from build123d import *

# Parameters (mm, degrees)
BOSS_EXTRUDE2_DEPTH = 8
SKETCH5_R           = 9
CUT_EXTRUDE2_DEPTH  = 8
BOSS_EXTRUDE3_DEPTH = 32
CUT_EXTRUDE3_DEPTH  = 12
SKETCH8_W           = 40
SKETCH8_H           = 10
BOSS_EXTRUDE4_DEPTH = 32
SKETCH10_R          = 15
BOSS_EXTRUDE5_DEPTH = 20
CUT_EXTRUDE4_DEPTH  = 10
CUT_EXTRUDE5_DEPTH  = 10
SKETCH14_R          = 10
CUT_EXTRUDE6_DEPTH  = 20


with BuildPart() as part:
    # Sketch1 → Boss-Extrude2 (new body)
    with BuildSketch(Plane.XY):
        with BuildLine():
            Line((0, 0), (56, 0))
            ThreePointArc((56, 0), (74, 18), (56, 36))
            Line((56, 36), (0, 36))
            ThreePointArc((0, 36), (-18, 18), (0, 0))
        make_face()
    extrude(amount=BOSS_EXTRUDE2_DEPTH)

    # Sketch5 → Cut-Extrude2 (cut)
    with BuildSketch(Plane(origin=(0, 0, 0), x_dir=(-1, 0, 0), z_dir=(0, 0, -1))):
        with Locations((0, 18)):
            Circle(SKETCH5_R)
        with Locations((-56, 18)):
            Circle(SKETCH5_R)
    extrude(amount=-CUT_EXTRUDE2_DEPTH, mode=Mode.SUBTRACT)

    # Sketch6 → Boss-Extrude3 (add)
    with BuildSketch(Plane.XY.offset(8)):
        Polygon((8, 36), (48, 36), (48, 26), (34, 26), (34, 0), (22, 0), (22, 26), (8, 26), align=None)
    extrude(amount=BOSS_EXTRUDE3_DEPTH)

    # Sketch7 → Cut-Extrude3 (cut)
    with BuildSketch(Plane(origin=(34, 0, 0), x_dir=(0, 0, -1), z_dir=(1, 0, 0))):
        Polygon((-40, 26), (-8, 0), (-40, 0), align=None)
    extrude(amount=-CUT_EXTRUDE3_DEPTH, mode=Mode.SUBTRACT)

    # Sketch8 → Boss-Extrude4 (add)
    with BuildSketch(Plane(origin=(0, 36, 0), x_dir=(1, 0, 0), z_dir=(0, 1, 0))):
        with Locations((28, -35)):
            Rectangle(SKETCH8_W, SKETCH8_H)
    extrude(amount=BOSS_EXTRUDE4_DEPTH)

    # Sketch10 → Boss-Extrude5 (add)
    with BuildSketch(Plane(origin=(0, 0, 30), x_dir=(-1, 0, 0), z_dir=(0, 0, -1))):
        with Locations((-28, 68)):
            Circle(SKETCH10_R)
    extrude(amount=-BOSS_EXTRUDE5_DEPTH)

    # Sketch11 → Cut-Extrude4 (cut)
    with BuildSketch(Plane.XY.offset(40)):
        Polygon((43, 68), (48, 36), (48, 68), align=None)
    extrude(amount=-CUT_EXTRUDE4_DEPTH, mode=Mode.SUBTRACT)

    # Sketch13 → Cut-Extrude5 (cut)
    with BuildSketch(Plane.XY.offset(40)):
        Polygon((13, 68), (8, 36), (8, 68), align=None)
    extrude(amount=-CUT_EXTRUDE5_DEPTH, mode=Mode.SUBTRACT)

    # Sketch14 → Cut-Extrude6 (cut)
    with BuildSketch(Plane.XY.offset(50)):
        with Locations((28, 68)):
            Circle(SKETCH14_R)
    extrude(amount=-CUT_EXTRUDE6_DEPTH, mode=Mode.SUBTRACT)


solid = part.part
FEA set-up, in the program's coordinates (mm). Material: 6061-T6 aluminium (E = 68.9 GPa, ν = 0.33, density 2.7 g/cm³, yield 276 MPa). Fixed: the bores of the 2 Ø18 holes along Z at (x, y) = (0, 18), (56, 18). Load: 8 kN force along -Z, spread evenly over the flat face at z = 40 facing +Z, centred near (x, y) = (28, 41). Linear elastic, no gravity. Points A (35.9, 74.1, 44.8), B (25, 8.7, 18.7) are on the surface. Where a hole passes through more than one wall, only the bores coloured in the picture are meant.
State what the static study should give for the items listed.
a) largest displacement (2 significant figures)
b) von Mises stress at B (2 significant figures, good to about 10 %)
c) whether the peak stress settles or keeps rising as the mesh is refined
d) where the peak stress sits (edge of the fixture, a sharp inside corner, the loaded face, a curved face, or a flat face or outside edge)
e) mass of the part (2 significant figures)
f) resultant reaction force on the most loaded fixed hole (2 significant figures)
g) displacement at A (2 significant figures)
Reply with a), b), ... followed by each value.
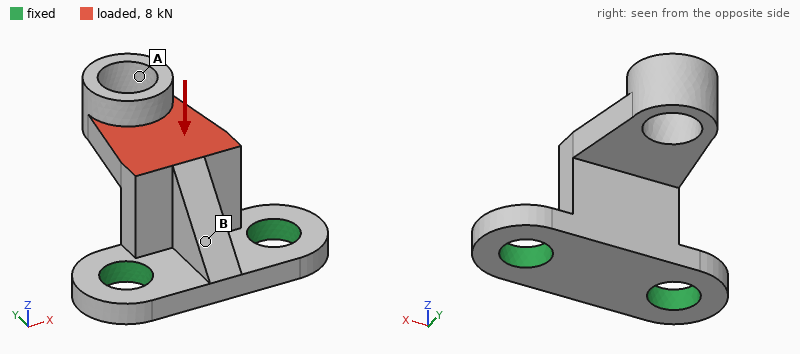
a) 0.55 mm
b) 43 MPa
c) keeps rising
d) edge of the fixture
e) 140 g
f) 4.4 kN
g) 0.46 mm
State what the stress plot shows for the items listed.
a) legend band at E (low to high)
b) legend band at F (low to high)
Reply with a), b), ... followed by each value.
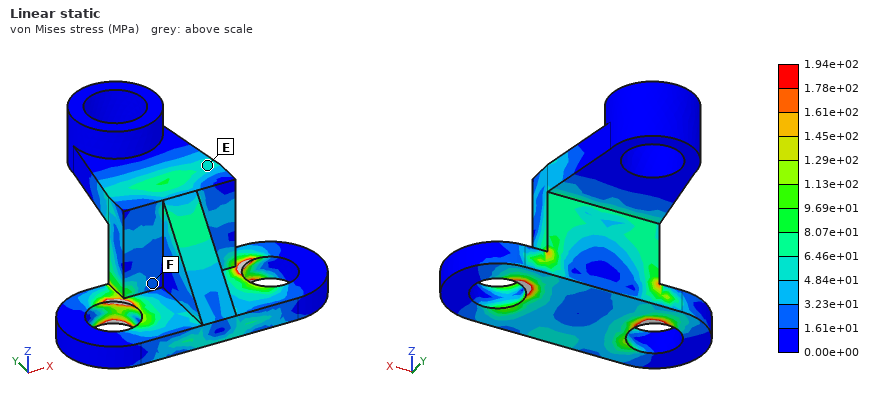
a) 4.84e+01 to 6.46e+01 MPa
b) 1.61e+01 to 3.23e+01 MPa
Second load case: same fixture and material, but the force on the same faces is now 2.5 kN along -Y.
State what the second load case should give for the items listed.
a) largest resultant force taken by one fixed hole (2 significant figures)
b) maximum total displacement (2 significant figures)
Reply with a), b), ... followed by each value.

a) 1.3 kN
b) 0.25 mm
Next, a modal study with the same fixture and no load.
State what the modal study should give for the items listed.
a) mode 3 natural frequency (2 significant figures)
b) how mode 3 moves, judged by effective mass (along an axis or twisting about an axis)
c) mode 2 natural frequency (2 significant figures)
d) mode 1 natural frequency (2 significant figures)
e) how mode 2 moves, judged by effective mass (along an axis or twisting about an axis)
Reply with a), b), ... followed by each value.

a) 5200 Hz
b) along Y
c) 3300 Hz
d) 2100 Hz
e) along X
